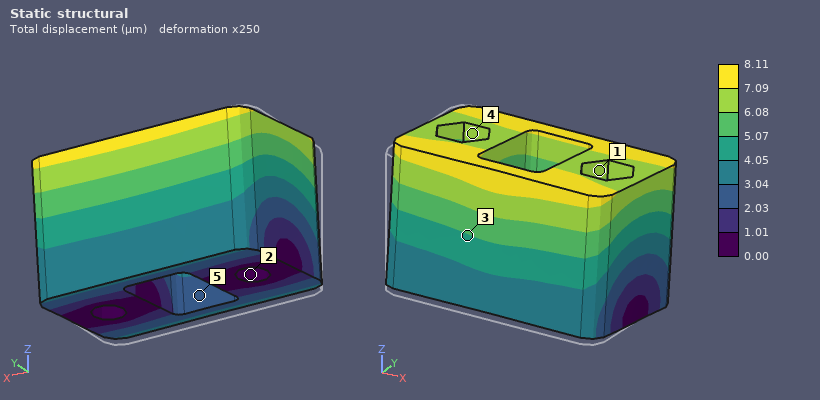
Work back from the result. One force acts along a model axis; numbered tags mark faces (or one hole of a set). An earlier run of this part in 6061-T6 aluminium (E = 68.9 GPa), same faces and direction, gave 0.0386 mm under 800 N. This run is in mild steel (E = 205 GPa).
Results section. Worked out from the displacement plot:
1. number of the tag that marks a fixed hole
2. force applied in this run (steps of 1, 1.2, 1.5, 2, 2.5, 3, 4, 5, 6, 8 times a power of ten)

2
500 N
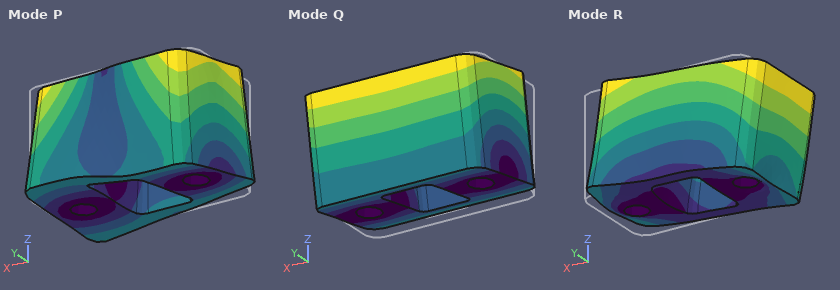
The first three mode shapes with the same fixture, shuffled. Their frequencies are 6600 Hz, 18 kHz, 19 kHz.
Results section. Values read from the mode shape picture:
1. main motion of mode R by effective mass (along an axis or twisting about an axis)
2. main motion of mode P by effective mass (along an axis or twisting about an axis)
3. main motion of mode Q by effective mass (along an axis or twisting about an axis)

along X
twisting about Z
along Y
